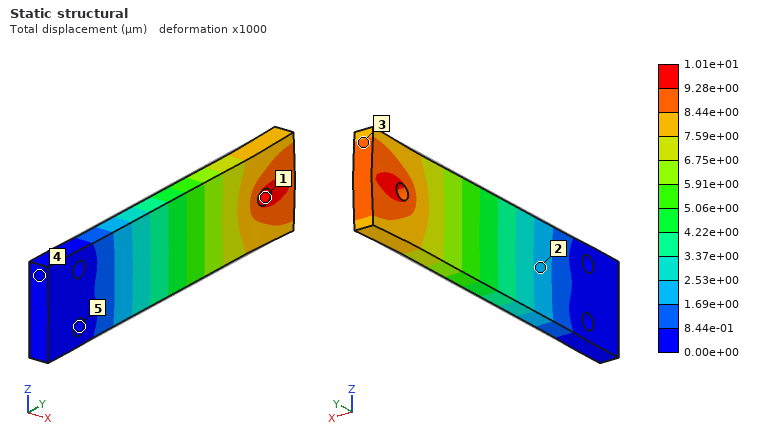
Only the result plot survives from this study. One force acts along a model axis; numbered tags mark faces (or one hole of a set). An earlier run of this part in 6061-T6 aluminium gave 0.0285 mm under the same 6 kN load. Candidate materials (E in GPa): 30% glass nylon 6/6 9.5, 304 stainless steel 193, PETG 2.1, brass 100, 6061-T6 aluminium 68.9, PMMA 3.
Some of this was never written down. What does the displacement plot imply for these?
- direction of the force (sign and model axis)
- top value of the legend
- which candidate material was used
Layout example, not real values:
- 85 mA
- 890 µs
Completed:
- +Y
- 1.01e+01 µm
- 304 stainless steel
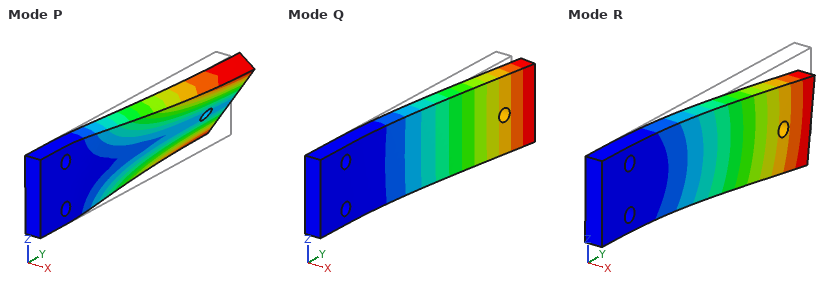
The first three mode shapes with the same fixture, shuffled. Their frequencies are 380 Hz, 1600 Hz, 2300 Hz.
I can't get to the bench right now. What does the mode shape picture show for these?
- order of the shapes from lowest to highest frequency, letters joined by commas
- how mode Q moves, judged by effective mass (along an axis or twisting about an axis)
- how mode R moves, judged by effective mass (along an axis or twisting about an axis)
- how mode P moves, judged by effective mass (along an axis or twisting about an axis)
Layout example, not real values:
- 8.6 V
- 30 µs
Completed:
- Q, R, P
- along X
- along Z
- twisting about Y
